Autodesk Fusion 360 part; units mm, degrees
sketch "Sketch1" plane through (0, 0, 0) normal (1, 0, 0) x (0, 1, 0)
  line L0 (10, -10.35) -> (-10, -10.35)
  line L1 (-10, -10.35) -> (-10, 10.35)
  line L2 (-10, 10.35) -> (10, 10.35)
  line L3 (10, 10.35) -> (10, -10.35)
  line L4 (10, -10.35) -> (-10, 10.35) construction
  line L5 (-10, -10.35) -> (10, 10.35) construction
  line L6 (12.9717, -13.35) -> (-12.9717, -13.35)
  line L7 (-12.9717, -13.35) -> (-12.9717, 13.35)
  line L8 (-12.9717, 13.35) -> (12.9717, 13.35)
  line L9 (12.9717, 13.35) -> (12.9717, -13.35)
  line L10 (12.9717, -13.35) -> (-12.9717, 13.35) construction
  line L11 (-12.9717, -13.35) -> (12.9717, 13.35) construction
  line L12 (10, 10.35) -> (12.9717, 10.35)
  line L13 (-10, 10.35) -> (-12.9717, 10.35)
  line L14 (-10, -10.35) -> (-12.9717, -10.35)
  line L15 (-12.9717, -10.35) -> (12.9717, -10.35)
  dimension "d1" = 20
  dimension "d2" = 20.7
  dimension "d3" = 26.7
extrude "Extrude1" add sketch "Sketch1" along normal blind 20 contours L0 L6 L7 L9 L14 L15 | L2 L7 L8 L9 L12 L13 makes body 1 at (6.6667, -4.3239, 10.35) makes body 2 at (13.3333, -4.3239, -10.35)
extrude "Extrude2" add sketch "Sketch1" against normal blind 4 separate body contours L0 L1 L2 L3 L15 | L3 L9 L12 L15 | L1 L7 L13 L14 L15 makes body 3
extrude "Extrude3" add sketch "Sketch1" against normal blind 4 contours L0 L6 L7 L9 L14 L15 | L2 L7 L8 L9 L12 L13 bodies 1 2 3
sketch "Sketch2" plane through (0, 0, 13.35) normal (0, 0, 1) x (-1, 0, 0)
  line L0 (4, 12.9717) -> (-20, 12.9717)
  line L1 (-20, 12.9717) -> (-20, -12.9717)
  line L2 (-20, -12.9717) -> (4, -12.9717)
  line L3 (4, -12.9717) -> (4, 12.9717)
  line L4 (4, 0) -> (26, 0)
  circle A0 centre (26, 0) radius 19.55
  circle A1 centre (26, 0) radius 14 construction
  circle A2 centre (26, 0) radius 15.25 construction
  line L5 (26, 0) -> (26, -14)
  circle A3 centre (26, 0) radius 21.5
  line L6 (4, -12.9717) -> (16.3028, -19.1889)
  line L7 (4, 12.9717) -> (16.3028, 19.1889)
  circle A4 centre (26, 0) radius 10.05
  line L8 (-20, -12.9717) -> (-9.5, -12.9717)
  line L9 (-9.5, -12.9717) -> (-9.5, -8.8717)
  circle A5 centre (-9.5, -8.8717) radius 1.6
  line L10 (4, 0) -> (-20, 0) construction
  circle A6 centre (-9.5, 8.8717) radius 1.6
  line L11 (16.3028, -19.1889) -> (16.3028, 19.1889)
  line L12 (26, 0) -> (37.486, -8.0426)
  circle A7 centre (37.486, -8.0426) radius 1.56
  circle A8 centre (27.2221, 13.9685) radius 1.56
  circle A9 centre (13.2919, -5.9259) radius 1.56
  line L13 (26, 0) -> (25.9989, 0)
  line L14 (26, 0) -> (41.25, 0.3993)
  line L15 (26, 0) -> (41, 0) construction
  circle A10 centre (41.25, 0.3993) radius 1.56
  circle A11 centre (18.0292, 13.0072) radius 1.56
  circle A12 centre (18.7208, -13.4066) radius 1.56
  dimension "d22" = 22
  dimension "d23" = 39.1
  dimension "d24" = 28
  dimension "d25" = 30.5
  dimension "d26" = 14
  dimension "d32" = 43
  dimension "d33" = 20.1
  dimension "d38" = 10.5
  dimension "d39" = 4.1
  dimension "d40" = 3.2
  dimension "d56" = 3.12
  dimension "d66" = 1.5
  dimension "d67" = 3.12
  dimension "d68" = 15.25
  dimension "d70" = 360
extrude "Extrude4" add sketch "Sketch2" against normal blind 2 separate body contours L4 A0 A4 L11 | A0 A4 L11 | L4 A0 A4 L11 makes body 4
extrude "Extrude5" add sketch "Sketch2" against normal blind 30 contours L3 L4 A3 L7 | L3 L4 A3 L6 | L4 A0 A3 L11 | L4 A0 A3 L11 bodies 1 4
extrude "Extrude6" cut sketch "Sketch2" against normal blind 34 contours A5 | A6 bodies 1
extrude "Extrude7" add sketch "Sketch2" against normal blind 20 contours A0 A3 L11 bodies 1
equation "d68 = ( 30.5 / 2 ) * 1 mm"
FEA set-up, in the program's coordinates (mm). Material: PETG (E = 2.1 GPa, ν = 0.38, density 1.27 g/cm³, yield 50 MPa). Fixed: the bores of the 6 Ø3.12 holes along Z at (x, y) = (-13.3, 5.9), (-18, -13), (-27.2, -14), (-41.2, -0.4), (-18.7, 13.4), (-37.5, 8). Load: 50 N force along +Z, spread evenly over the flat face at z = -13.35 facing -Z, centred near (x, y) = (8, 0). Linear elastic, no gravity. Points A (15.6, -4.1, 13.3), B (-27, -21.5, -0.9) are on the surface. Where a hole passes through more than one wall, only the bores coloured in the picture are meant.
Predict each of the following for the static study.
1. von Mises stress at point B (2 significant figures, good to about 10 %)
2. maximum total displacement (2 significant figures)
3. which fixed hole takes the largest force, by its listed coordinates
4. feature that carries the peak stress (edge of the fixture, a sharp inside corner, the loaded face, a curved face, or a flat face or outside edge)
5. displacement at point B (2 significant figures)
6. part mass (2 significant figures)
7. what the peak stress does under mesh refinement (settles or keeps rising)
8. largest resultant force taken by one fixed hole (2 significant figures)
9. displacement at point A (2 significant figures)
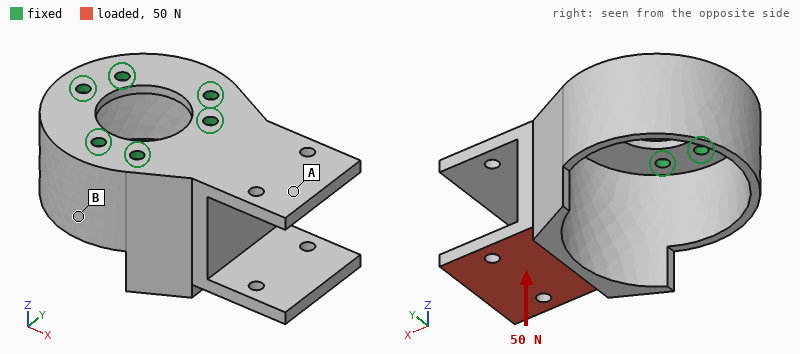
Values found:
2.0 MPa
0.86 mm
(-13.3, 5.9)
edge of the fixture
0.14 mm
20 g
keeps rising
55 N
0.30 mm
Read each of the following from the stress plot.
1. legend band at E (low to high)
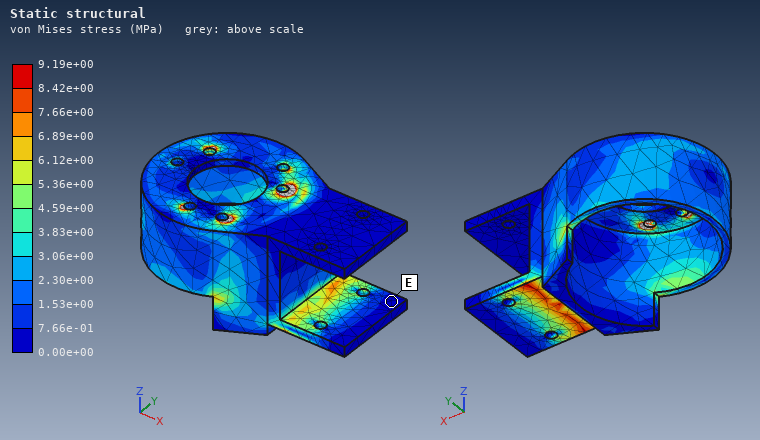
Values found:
0.00e+00 to 7.66e-01 MPa
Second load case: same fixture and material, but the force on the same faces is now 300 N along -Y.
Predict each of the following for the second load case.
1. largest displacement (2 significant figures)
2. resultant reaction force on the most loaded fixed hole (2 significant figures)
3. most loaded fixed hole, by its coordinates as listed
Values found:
0.83 mm
280 N
(-18, -13)
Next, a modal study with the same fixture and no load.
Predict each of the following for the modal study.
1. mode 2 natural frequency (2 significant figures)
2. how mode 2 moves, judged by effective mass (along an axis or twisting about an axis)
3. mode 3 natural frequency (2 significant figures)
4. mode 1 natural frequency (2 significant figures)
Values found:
1200 Hz
along Y
1300 Hz
620 Hz
